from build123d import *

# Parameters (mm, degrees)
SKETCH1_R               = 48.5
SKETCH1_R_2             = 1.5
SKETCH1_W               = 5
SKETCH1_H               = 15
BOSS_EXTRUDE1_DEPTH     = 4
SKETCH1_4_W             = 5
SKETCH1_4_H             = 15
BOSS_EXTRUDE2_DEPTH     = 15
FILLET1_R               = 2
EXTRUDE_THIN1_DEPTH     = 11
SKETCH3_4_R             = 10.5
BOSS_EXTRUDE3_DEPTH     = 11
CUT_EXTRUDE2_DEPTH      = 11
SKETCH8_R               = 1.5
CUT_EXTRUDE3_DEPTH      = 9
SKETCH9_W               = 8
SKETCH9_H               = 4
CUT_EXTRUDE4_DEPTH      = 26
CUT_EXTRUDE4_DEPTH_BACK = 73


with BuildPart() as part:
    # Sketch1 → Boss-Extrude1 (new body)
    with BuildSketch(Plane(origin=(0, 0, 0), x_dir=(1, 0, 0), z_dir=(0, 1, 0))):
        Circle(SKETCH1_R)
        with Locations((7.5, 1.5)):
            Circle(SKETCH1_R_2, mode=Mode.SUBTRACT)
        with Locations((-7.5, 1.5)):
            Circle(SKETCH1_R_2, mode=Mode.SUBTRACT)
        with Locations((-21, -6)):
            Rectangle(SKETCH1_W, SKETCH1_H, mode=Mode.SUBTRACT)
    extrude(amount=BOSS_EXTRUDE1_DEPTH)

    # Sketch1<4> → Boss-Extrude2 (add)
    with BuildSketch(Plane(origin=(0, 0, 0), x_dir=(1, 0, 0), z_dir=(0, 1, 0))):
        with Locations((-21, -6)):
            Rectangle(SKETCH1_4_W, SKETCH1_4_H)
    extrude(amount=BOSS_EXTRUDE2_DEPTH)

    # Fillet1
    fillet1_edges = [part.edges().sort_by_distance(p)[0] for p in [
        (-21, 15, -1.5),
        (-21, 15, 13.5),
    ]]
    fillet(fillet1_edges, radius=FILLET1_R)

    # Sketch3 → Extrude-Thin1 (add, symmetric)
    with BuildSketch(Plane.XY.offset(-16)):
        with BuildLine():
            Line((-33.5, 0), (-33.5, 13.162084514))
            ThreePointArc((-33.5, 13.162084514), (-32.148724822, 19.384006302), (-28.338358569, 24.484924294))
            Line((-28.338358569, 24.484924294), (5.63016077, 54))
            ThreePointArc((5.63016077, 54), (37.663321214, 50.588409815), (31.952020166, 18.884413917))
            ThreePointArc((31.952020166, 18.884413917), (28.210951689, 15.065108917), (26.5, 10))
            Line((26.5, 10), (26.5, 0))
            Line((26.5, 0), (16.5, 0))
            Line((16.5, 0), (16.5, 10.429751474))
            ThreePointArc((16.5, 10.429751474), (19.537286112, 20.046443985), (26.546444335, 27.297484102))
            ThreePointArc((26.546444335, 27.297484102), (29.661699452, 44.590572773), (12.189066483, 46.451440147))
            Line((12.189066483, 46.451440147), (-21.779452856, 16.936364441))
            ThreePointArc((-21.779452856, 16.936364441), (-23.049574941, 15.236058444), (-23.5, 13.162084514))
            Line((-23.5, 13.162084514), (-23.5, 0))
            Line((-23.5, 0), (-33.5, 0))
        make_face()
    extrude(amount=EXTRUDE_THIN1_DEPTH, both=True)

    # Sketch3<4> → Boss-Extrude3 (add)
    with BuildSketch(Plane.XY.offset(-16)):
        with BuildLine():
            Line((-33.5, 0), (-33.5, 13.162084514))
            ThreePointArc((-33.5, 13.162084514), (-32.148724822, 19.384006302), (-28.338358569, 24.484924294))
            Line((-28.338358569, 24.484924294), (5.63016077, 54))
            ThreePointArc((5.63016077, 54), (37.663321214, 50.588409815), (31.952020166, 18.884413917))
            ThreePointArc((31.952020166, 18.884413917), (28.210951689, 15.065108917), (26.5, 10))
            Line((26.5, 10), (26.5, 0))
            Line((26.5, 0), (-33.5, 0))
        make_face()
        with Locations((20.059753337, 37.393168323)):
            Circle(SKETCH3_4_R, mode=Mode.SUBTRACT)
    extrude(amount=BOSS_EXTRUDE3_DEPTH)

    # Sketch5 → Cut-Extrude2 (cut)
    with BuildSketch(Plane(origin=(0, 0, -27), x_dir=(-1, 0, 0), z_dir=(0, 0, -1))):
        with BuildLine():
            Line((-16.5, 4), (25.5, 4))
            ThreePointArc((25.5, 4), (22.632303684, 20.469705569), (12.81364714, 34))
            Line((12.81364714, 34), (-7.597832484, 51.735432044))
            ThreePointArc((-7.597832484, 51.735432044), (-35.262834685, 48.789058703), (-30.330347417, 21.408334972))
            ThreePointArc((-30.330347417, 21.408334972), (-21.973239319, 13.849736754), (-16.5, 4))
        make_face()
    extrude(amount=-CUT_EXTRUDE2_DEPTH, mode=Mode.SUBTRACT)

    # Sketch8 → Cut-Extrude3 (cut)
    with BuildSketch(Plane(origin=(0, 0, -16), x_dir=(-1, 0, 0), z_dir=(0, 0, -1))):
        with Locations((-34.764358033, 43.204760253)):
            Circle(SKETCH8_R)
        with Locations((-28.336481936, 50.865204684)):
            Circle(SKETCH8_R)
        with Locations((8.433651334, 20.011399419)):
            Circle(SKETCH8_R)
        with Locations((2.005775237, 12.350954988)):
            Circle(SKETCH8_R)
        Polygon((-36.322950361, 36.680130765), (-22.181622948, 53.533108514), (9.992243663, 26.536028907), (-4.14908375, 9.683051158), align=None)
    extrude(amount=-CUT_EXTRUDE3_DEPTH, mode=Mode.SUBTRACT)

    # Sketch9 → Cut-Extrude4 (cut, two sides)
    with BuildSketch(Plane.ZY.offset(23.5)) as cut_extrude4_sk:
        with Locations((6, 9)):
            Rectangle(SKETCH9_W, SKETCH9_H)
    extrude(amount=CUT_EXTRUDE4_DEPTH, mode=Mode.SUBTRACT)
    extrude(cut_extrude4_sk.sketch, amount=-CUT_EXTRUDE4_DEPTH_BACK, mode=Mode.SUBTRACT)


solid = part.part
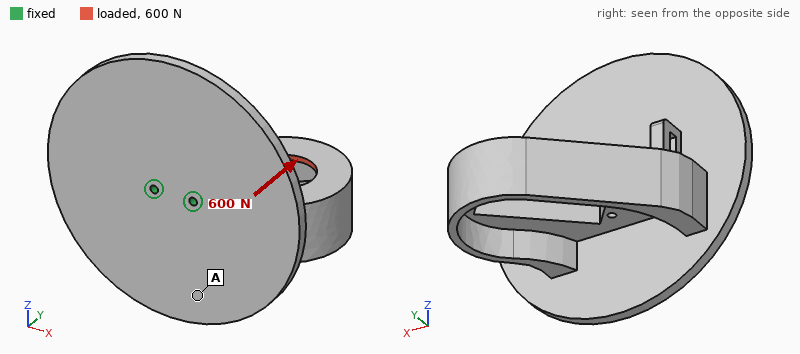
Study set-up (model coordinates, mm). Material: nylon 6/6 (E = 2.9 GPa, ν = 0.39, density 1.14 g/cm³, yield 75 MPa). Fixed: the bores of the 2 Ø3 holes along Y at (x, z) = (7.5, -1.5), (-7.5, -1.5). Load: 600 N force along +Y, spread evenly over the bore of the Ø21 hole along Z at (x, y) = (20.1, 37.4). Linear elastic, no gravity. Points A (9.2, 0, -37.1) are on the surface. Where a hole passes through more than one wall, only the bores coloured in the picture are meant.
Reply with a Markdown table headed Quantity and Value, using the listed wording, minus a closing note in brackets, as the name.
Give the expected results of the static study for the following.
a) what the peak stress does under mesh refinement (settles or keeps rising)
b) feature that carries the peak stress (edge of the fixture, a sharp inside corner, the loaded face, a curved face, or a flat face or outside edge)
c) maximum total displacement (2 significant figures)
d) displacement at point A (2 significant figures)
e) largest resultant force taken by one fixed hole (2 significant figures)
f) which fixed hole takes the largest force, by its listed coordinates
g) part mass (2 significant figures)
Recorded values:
| Quantity | Value |
|---|---|
| what the peak stress does under mesh refinement | keeps rising |
| feature that carries the peak stress | edge of the fixture |
| maximum total displacement | 1.5 mm |
| displacement at point A | 0.67 mm |
| largest resultant force taken by one fixed hole | 930 N |
| which fixed hole takes the largest force, by its listed coordinates | (7.5, -1.5) |
| part mass | 68 g |
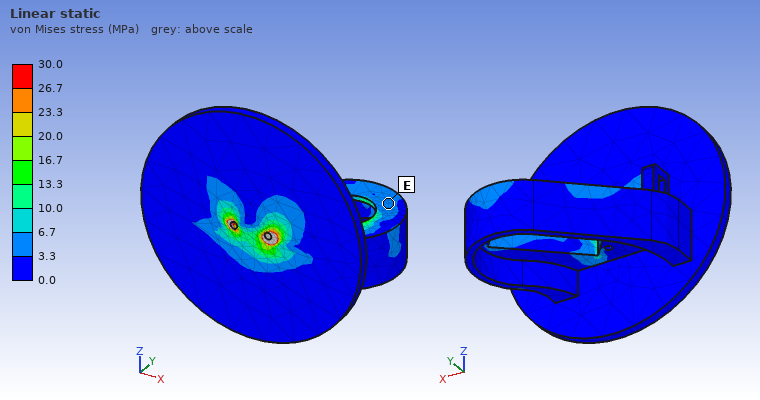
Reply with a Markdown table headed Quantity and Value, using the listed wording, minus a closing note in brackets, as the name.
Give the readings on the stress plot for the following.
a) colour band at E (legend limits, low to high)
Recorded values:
| Quantity | Value |
|---|---|
| colour band at E | 3.3 to 6.7 MPa |
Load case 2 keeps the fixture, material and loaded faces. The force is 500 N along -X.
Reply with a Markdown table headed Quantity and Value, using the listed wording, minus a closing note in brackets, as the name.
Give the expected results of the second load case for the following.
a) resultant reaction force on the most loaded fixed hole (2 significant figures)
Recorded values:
| Quantity | Value |
|---|---|
| resultant reaction force on the most loaded fixed hole | 980 N |
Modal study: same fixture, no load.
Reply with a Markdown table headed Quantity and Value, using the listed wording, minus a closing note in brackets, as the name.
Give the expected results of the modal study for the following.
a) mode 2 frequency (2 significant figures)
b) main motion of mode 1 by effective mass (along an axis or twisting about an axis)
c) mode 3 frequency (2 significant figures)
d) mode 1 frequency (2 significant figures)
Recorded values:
| Quantity | Value |
|---|---|
| mode 2 frequency | 520 Hz |
| main motion of mode 1 by effective mass | along Z |
| mode 3 frequency | 530 Hz |
| mode 1 frequency | 250 Hz |
